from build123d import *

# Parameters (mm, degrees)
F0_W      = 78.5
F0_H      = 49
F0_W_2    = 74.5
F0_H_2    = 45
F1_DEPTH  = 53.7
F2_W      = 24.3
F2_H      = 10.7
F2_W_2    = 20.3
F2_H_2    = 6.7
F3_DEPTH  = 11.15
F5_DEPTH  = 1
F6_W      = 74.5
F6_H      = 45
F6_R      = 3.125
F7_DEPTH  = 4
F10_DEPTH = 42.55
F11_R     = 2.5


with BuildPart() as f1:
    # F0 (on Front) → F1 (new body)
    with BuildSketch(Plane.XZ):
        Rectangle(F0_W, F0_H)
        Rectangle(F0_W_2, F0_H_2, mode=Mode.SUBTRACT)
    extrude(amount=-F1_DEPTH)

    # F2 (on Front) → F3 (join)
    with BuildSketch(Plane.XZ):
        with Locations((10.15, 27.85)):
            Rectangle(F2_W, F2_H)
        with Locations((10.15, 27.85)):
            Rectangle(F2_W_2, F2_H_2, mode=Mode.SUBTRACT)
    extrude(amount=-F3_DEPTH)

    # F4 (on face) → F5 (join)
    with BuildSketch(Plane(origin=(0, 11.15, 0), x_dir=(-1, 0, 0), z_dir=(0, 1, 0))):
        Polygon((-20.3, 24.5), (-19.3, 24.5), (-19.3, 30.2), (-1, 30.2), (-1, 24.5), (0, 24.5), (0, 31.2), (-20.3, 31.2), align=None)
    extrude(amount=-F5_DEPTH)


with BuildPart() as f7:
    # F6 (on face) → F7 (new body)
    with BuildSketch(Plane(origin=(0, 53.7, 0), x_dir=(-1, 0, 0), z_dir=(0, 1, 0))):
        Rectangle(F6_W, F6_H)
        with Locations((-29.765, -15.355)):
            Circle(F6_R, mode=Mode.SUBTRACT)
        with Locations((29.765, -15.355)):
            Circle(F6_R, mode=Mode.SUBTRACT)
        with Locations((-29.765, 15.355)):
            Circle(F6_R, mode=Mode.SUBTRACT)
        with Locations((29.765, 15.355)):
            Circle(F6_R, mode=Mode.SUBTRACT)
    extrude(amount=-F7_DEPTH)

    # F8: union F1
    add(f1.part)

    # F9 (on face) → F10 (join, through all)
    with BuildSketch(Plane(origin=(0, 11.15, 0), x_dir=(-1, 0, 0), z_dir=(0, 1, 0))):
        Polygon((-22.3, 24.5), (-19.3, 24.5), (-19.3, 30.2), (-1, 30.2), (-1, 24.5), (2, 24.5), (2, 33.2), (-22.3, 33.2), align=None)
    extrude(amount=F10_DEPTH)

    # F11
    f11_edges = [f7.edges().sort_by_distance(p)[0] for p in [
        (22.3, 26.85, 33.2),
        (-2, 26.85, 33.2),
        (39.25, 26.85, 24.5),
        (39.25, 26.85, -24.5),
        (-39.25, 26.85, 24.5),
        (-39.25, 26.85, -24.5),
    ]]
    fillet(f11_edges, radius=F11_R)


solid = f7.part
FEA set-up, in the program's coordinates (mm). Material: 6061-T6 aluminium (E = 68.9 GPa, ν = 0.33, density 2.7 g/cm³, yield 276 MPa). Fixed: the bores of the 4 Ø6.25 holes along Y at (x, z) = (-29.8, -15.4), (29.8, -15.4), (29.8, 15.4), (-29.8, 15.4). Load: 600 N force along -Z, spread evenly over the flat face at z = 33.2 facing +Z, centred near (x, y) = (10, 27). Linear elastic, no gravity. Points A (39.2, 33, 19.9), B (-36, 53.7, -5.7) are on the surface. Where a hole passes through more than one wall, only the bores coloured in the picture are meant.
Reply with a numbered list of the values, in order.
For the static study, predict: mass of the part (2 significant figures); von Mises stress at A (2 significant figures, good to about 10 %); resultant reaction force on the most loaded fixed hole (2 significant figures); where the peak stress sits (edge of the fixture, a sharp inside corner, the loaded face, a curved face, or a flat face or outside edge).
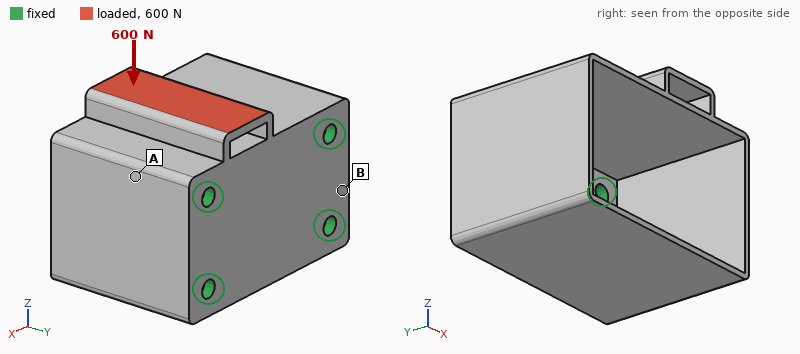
1. 120 g
2. 24 MPa
3. 360 N
4. a flat face or outside edge
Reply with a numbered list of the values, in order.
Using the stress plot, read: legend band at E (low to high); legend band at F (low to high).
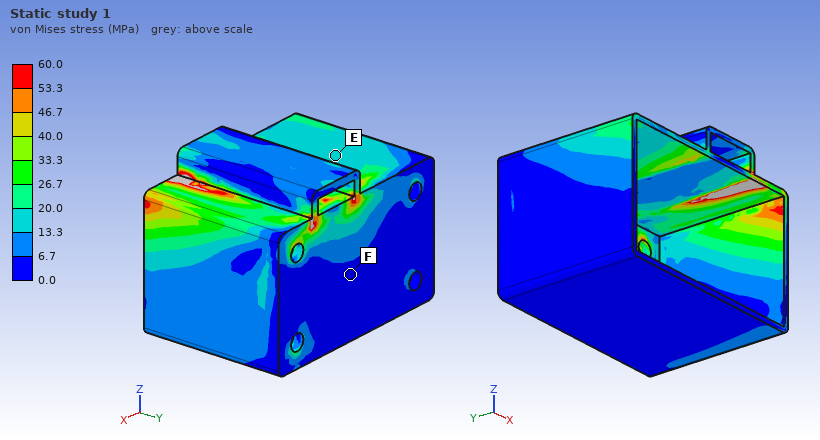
1. 13.3 to 20.0 MPa
2. 0.0 to 6.7 MPa
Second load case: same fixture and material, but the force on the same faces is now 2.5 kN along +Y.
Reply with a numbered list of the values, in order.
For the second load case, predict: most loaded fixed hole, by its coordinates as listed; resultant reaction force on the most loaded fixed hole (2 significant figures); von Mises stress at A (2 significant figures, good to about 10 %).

1. (29.8, 15.4)
2. 2.4 kN
3. 51 MPa
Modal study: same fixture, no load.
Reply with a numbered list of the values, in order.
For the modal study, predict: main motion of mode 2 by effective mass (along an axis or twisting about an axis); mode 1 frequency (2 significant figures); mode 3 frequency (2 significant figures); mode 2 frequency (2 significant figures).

1. along Z
2. 1700 Hz
3. 3300 Hz
4. 1900 Hz
